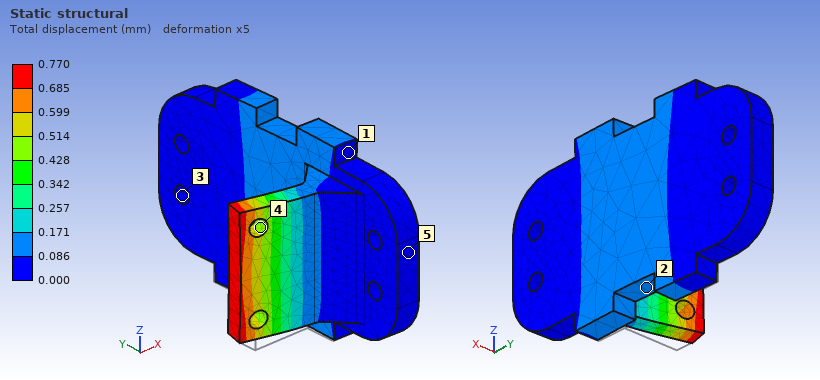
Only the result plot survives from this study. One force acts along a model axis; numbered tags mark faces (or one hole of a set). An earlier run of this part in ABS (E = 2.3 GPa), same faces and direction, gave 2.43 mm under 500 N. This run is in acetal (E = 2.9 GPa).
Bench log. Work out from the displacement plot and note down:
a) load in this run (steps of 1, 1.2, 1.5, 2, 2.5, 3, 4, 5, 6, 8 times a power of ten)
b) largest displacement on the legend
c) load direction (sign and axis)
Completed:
200 N
0.770 mm
+Y
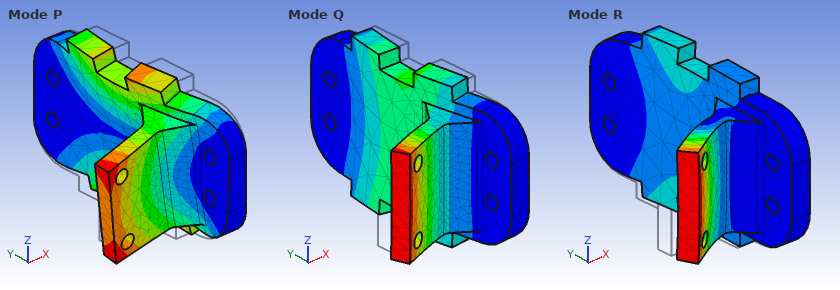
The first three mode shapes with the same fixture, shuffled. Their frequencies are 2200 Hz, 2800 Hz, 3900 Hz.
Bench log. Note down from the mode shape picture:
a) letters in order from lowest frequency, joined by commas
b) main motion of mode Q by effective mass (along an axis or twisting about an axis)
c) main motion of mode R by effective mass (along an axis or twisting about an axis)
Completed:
Q, P, R
along X
along X
